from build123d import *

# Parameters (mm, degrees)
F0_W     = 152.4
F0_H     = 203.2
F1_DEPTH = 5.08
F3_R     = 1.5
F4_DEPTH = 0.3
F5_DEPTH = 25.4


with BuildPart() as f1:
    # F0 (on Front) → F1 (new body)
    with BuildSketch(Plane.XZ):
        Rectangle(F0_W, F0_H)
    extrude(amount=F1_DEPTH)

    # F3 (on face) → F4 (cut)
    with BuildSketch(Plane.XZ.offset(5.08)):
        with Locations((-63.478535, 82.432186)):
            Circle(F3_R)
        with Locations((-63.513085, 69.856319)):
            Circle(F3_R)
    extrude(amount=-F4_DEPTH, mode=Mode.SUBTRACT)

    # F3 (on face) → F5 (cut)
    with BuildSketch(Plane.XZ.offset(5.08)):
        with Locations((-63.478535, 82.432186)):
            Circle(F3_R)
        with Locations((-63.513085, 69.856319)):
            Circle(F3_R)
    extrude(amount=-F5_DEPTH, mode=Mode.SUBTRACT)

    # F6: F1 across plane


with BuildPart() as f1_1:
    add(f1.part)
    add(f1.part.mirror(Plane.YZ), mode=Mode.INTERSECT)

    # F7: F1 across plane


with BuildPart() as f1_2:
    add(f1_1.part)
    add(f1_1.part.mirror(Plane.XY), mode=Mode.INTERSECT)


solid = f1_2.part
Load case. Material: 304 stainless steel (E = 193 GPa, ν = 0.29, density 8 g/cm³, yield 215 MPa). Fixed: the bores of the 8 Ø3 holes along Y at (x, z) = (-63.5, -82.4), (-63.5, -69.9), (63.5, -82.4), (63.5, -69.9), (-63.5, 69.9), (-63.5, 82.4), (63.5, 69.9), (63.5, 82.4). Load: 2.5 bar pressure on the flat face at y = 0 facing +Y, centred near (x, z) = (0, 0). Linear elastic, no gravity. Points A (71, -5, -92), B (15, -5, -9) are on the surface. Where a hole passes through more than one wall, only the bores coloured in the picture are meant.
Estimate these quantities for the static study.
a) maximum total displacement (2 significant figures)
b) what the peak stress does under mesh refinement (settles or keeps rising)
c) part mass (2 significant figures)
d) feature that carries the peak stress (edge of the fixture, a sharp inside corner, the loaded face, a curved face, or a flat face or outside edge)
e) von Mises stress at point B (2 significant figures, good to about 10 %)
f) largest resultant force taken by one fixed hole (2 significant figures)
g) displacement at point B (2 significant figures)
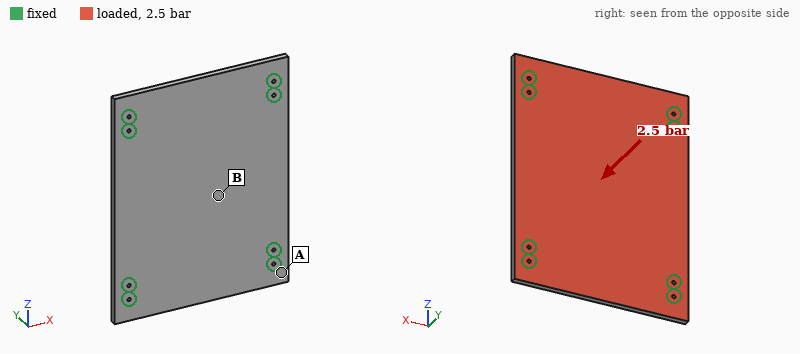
0.29 mm
keeps rising
1.3 kg
edge of the fixture
55 MPa
2.2 kN
0.28 mm
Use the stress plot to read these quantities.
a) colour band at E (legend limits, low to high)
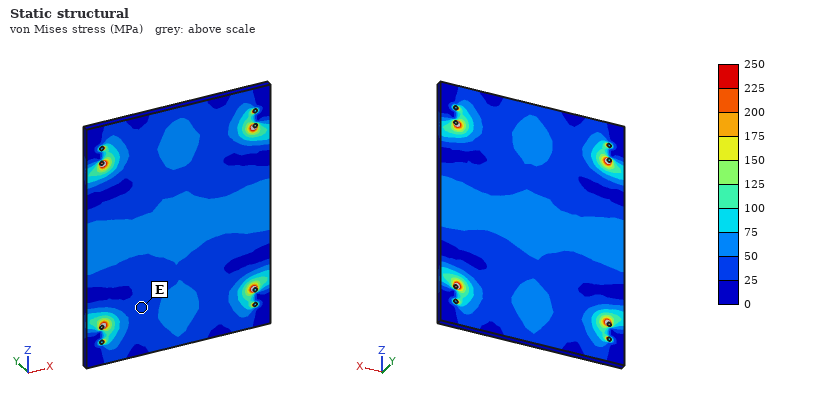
25 to 50 MPa
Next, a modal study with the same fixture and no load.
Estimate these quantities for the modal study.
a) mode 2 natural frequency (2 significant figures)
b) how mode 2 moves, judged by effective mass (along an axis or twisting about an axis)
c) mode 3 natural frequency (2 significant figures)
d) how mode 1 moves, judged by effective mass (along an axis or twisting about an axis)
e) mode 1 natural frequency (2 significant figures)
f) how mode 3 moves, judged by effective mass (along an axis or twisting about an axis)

1400 Hz
twisting about Z
1500 Hz
along Y
890 Hz
twisting about X
